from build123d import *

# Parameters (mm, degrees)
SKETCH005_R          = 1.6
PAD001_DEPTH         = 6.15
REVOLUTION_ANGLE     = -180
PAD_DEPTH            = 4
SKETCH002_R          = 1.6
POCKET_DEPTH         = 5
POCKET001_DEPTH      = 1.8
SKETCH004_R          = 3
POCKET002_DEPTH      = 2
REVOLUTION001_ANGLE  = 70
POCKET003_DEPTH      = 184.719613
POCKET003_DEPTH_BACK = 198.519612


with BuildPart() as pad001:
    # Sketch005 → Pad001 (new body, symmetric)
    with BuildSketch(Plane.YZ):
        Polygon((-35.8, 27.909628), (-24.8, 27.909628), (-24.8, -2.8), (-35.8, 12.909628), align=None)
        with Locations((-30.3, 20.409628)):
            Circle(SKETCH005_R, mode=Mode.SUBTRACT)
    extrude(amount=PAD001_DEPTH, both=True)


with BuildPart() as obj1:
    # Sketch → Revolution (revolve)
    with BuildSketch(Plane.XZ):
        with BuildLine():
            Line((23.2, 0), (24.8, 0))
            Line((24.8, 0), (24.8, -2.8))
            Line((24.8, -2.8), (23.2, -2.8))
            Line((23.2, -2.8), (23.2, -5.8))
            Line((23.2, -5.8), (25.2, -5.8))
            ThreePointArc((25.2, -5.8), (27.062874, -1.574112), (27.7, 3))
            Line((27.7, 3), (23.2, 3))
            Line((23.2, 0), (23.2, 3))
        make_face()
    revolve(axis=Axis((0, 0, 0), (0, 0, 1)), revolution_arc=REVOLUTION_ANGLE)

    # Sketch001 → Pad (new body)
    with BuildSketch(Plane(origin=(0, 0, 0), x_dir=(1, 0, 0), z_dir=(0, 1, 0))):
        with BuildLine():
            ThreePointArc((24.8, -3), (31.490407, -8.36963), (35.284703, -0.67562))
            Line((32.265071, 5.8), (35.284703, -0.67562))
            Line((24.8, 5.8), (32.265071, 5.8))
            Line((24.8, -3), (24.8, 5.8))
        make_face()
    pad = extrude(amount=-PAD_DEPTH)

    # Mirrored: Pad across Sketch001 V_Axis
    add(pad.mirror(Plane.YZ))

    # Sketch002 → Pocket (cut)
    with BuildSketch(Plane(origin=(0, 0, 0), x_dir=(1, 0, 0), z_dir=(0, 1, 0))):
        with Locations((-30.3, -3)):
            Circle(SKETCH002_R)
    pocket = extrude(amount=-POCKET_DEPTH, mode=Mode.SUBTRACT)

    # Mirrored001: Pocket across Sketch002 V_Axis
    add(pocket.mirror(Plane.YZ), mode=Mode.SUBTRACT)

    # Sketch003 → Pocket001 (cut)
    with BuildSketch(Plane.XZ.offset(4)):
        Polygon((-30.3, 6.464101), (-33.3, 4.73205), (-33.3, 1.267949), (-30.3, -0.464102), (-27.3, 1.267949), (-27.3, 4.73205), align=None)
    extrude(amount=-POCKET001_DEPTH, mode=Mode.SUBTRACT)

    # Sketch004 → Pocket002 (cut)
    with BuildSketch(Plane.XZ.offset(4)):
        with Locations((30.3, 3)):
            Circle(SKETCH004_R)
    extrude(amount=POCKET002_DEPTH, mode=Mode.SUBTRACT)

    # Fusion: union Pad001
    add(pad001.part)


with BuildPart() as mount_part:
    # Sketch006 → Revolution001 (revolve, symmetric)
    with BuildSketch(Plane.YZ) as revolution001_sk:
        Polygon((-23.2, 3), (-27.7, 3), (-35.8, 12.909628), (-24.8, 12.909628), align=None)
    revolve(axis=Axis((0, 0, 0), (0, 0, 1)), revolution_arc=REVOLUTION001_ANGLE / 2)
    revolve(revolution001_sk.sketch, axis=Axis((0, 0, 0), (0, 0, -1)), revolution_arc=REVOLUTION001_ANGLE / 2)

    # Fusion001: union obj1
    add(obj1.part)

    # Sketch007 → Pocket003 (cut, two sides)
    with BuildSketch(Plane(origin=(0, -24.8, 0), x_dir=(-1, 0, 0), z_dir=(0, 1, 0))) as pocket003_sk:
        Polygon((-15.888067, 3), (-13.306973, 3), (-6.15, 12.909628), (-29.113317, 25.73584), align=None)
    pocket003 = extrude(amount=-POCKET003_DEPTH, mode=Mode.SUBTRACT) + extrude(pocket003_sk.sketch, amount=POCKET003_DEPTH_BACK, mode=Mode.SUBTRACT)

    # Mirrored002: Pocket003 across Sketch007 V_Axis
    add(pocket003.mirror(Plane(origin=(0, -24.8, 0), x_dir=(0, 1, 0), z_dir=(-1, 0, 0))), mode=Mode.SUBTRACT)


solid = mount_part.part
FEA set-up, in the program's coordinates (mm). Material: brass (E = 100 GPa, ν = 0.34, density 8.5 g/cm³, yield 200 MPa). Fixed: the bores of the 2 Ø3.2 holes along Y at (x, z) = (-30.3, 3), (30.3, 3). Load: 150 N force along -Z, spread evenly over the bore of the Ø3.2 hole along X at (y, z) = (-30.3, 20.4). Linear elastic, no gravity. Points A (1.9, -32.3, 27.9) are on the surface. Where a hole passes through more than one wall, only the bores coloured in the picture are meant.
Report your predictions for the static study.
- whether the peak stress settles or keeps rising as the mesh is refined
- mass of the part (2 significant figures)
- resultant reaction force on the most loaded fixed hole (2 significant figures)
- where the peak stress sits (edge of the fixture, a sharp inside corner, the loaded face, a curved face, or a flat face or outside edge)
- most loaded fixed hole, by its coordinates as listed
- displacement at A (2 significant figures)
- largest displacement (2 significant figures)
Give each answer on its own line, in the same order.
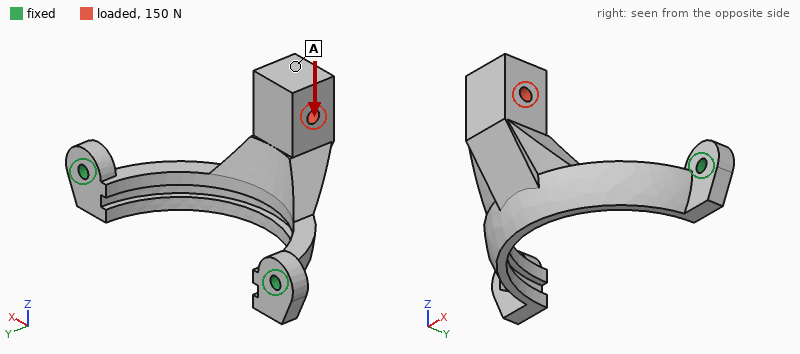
keeps rising
55 g
83 N
edge of the fixture
(30.3, 3)
0.21 mm
0.22 mm
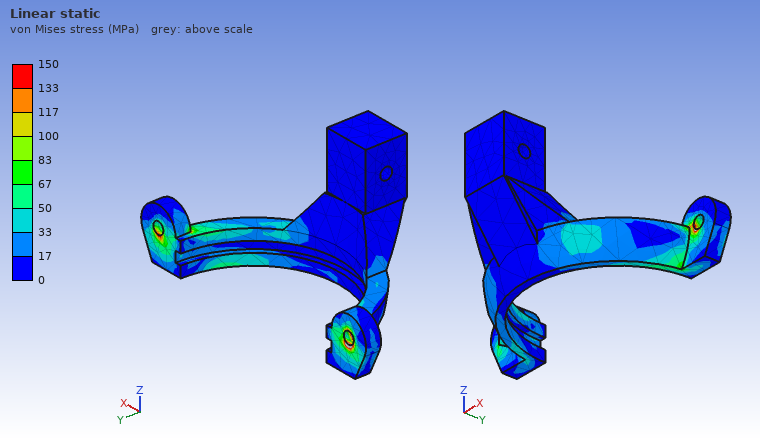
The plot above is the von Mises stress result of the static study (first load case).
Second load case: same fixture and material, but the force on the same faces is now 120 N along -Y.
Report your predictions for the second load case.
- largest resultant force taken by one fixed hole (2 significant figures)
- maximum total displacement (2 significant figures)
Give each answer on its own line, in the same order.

74 N
0.19 mm
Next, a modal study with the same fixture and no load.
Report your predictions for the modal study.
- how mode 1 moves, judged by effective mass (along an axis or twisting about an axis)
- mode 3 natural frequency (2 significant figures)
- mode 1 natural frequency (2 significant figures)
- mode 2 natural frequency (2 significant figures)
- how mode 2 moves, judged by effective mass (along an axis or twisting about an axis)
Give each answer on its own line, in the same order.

along Z
2500 Hz
780 Hz
2100 Hz
along X
